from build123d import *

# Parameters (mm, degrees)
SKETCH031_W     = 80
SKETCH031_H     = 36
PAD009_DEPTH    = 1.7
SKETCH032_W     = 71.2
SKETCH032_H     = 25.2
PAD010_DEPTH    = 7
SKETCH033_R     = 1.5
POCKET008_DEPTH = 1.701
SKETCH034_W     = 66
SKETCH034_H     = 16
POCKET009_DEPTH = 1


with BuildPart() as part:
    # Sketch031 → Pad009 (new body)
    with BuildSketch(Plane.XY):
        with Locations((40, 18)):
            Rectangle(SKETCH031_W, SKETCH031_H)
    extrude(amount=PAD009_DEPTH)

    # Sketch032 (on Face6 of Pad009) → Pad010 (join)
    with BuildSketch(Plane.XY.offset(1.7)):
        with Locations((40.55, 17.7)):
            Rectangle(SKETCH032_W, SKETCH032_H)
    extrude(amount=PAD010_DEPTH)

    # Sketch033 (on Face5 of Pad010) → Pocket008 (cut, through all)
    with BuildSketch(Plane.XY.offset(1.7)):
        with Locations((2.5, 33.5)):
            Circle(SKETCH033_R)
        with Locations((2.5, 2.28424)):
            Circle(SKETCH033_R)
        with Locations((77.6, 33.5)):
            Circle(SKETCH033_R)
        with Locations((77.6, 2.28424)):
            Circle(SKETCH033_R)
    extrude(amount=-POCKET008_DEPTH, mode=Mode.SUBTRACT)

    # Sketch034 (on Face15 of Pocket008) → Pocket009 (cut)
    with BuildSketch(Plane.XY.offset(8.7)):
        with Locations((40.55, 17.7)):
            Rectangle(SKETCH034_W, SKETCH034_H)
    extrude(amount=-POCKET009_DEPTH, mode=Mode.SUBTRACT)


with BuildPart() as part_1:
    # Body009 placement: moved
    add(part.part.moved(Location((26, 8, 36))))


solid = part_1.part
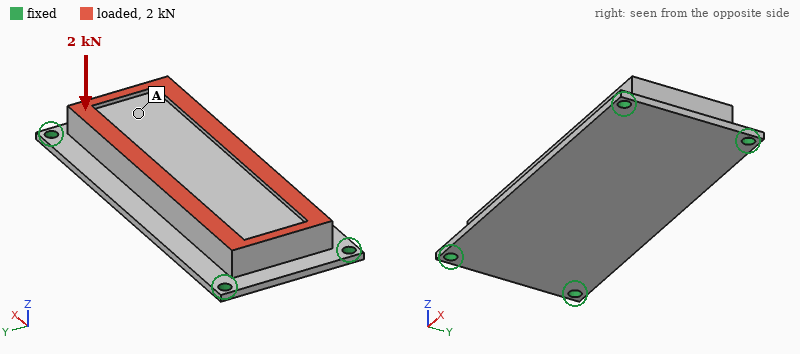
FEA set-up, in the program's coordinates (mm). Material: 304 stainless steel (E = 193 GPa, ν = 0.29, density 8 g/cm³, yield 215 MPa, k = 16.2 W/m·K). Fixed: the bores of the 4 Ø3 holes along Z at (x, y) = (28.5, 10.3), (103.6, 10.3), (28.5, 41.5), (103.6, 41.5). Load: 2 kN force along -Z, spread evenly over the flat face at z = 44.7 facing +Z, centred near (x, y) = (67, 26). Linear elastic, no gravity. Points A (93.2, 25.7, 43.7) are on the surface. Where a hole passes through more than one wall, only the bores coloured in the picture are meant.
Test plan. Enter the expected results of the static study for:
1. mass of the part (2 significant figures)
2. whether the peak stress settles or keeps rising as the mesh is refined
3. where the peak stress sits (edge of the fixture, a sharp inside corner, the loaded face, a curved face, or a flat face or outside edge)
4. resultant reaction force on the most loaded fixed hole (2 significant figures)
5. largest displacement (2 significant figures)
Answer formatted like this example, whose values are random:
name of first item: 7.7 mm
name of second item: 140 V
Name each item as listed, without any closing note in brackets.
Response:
mass of the part: 130 g
whether the peak stress settles or keeps rising as the mesh is refined: keeps rising
where the peak stress sits: edge of the fixture
resultant reaction force on the most loaded fixed hole: 920 N
largest displacement: 37 µm
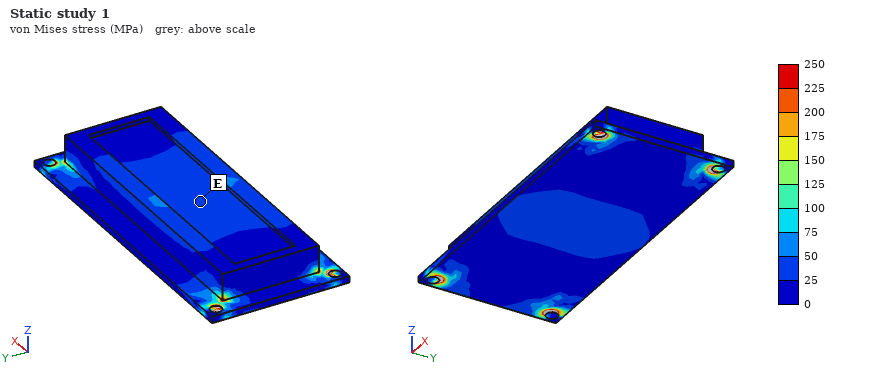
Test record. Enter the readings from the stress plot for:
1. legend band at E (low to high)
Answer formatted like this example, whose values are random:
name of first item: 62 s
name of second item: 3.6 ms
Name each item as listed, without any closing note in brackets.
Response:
legend band at E: 25 to 50 MPa
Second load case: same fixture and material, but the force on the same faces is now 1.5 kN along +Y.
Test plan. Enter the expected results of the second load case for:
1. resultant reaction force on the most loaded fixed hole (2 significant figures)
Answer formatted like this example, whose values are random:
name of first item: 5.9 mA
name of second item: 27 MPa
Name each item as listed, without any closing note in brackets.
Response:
resultant reaction force on the most loaded fixed hole: 530 N
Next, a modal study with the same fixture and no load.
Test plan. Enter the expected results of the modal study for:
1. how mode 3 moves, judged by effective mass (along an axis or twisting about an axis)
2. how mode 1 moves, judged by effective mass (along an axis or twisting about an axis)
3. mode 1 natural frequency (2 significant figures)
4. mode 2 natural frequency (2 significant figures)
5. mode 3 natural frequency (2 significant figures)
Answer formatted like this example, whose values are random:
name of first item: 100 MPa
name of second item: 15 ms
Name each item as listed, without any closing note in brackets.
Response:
how mode 3 moves, judged by effective mass: twisting about Y
how mode 1 moves, judged by effective mass: along Z
mode 1 natural frequency: 3700 Hz
mode 2 natural frequency: 7300 Hz
mode 3 natural frequency: 8900 Hz
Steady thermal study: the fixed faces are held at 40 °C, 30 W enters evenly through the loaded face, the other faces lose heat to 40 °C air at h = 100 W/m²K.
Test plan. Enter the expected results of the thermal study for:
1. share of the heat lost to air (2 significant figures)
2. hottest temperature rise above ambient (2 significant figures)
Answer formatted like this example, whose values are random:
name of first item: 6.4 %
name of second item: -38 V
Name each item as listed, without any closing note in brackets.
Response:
share of the heat lost to air: 82 %
hottest temperature rise above ambient: 52 K
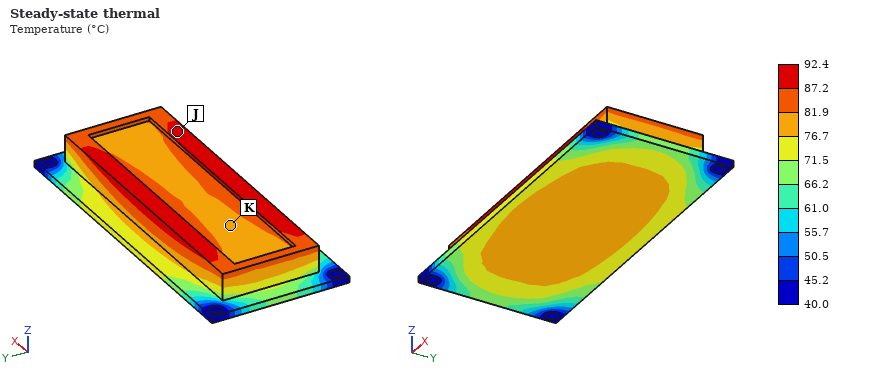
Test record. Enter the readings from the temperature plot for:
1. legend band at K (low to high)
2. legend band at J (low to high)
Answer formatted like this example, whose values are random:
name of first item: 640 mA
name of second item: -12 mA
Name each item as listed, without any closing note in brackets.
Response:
legend band at K: 76.7 to 81.9 °C
legend band at J: 87.2 to 92.4 °C
